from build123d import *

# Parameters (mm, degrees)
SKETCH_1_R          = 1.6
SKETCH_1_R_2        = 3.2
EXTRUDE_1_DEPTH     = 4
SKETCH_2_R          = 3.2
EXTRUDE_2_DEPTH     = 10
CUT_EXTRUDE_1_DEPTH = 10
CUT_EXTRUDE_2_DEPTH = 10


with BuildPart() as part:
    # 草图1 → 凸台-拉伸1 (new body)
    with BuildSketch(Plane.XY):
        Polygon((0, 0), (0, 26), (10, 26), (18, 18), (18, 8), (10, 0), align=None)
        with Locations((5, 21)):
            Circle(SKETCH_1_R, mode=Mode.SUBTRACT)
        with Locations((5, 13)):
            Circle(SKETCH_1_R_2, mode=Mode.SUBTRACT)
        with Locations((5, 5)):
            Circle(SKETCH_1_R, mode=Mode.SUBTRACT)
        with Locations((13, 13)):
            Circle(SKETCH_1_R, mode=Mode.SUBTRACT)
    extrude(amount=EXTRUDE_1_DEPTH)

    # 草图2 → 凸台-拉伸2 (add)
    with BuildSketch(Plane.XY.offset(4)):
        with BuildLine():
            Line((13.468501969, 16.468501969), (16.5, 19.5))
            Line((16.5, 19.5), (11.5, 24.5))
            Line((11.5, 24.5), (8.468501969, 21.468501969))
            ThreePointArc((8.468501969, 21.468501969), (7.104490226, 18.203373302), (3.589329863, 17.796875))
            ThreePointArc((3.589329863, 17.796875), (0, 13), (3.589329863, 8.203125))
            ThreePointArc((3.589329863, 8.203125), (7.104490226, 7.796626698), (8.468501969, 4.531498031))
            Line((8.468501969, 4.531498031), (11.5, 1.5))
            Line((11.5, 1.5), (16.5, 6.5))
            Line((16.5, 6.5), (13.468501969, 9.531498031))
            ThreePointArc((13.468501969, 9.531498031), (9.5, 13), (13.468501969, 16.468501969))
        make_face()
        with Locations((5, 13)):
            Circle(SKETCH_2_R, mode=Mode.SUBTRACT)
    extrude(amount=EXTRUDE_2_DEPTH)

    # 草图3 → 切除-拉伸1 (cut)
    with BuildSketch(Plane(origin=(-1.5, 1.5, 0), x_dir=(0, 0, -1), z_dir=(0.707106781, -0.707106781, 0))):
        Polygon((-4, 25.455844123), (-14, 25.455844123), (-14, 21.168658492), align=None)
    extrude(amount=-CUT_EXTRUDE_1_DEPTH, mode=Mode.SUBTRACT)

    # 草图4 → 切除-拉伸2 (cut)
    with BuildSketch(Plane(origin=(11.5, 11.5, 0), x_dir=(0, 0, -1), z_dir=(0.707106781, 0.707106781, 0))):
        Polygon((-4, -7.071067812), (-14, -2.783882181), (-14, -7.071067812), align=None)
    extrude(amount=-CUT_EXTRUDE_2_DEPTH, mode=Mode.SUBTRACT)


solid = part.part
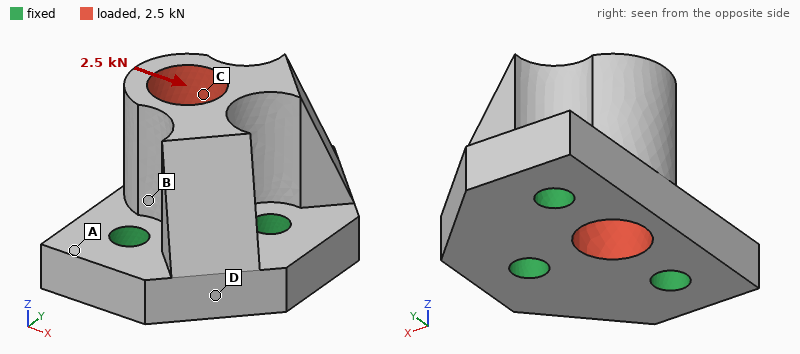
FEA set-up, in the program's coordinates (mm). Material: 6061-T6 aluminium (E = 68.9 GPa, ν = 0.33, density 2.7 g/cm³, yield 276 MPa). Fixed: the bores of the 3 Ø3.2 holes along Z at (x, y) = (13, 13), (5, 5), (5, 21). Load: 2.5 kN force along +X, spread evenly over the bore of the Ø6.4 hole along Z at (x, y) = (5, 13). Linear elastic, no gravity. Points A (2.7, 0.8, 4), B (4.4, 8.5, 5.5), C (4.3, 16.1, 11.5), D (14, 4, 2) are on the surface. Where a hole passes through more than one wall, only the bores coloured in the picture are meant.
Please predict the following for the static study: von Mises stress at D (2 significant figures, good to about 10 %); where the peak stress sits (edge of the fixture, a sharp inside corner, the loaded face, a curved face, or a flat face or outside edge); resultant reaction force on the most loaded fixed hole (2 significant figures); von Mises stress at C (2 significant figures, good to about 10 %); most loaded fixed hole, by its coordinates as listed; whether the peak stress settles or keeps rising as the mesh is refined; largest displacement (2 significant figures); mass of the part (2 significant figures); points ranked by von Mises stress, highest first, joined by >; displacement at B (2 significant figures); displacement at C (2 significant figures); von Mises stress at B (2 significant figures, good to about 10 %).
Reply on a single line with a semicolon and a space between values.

25 MPa; edge of the fixture; 1.4 kN; 48 MPa; (13, 13); keeps rising; 27 µm; 6.7 g; B > C > D > A; 9.1 µm; 20 µm; 67 MPa
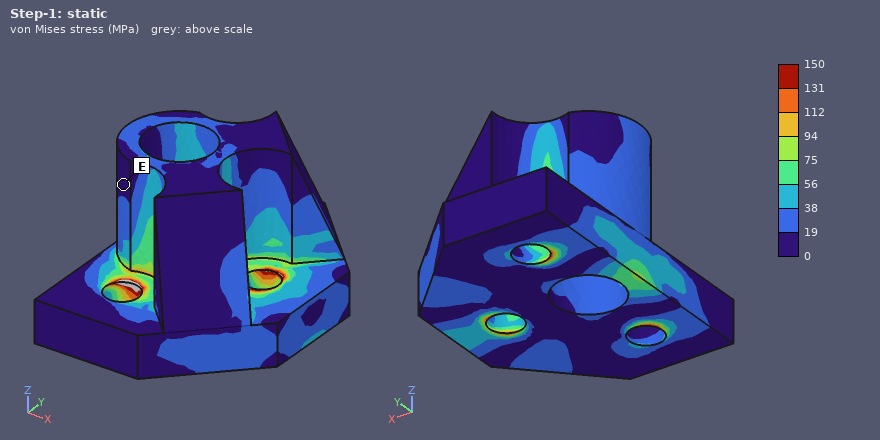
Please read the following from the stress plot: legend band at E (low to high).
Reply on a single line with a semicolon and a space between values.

0 to 19 MPa
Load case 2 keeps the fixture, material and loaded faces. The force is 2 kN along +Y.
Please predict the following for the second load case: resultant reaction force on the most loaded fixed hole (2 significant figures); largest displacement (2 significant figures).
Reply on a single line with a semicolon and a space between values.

990 N; 20 µm
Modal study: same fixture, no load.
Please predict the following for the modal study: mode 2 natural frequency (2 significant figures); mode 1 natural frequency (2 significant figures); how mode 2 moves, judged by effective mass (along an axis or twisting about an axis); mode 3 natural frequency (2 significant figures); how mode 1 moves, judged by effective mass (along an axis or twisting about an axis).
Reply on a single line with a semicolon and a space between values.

36 kHz; 31 kHz; along Y; 50 kHz; along X
